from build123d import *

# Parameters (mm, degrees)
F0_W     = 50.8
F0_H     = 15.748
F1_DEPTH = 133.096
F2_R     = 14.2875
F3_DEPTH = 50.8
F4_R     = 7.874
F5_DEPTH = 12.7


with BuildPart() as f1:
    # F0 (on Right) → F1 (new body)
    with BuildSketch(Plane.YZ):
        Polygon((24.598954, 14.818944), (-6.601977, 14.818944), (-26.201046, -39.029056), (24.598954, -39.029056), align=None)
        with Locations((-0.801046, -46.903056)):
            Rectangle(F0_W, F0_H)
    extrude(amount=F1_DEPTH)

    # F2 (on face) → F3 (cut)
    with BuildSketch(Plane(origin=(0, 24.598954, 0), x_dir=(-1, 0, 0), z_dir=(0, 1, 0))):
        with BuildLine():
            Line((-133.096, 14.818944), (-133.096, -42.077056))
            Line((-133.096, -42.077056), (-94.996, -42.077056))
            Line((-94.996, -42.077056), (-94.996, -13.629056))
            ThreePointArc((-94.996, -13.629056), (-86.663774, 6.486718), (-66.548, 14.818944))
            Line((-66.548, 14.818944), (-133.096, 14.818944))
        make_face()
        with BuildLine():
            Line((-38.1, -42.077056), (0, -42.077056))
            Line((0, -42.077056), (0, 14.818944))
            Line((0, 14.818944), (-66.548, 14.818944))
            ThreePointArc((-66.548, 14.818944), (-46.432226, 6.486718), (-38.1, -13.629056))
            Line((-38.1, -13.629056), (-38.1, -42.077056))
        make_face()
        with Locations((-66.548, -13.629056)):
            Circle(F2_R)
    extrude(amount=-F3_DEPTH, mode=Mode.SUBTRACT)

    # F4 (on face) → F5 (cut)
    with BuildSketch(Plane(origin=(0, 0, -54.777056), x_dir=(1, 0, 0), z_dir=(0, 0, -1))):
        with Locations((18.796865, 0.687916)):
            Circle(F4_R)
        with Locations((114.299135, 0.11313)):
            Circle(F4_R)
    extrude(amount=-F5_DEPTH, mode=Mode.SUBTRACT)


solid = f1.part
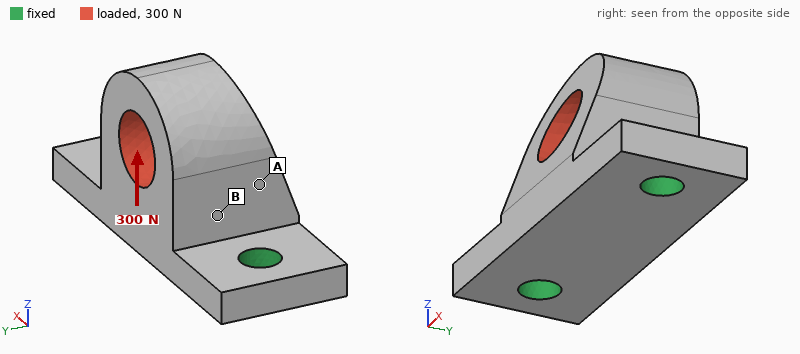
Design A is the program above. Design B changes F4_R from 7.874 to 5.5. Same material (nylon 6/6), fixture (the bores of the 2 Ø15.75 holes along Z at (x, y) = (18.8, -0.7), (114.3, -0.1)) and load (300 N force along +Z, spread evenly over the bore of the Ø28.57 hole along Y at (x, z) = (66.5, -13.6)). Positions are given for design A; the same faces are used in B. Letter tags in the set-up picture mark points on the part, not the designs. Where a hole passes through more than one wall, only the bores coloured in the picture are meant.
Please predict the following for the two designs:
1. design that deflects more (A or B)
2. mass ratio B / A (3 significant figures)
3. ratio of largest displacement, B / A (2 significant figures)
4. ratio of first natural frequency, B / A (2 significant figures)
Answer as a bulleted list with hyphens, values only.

- B
- 1.01
- 1.3
- 0.88
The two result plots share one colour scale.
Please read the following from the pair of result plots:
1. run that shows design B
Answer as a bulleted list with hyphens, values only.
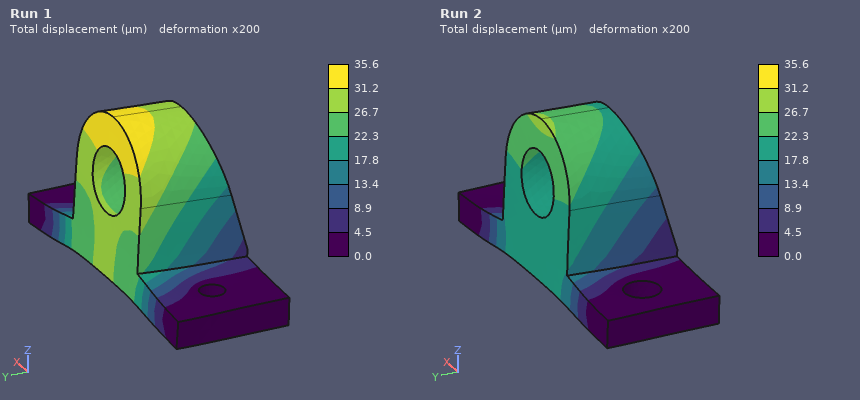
- Run 1
